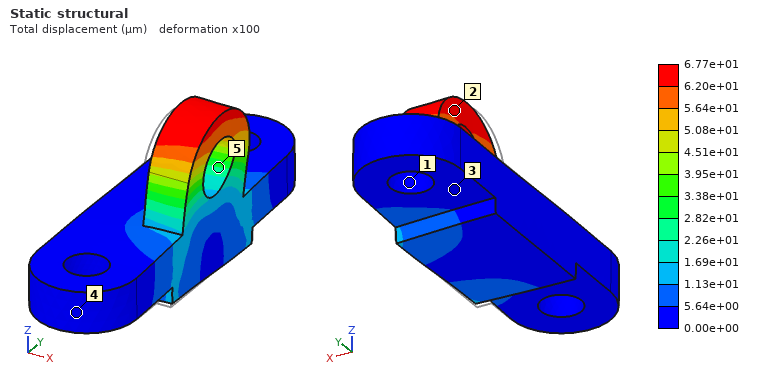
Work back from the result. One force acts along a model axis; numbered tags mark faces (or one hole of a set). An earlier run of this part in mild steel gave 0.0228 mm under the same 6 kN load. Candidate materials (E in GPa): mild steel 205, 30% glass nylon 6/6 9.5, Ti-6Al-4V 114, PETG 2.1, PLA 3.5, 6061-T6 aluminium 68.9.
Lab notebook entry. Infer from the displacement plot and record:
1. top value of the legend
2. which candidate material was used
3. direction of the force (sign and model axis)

6.77e+01 µm
6061-T6 aluminium
+Y
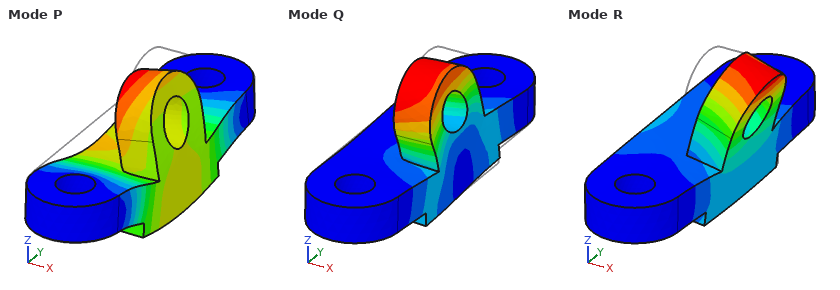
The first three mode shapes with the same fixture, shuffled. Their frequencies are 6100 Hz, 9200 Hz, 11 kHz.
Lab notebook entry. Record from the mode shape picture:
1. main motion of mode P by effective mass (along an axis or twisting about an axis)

along Z
